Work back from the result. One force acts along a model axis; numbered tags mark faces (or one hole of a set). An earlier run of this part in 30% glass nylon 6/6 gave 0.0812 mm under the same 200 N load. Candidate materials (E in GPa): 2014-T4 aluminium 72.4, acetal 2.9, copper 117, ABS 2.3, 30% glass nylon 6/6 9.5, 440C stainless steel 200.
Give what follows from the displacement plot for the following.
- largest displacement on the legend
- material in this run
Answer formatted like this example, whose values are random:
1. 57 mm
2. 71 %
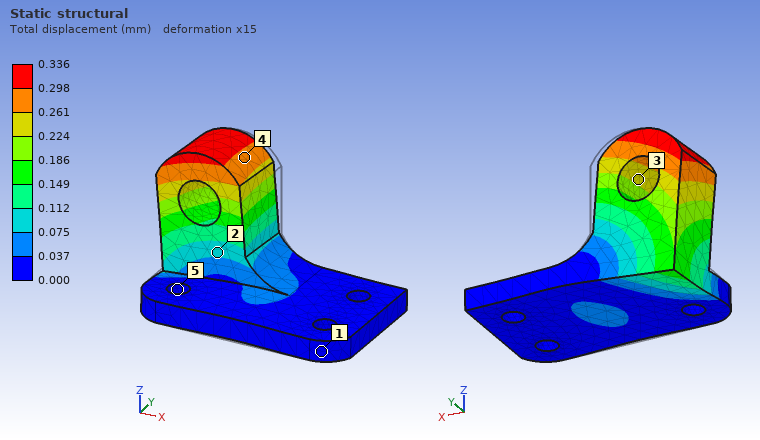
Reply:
1. 0.336 mm
2. ABS
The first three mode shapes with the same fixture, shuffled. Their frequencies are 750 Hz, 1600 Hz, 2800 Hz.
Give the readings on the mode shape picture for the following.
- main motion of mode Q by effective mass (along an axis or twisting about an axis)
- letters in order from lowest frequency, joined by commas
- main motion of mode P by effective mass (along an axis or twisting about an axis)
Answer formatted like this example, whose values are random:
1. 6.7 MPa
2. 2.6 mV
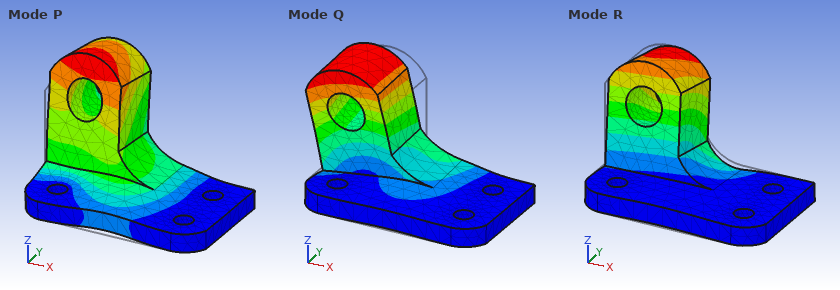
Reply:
1. along X
2. R, Q, P
3. along Z
